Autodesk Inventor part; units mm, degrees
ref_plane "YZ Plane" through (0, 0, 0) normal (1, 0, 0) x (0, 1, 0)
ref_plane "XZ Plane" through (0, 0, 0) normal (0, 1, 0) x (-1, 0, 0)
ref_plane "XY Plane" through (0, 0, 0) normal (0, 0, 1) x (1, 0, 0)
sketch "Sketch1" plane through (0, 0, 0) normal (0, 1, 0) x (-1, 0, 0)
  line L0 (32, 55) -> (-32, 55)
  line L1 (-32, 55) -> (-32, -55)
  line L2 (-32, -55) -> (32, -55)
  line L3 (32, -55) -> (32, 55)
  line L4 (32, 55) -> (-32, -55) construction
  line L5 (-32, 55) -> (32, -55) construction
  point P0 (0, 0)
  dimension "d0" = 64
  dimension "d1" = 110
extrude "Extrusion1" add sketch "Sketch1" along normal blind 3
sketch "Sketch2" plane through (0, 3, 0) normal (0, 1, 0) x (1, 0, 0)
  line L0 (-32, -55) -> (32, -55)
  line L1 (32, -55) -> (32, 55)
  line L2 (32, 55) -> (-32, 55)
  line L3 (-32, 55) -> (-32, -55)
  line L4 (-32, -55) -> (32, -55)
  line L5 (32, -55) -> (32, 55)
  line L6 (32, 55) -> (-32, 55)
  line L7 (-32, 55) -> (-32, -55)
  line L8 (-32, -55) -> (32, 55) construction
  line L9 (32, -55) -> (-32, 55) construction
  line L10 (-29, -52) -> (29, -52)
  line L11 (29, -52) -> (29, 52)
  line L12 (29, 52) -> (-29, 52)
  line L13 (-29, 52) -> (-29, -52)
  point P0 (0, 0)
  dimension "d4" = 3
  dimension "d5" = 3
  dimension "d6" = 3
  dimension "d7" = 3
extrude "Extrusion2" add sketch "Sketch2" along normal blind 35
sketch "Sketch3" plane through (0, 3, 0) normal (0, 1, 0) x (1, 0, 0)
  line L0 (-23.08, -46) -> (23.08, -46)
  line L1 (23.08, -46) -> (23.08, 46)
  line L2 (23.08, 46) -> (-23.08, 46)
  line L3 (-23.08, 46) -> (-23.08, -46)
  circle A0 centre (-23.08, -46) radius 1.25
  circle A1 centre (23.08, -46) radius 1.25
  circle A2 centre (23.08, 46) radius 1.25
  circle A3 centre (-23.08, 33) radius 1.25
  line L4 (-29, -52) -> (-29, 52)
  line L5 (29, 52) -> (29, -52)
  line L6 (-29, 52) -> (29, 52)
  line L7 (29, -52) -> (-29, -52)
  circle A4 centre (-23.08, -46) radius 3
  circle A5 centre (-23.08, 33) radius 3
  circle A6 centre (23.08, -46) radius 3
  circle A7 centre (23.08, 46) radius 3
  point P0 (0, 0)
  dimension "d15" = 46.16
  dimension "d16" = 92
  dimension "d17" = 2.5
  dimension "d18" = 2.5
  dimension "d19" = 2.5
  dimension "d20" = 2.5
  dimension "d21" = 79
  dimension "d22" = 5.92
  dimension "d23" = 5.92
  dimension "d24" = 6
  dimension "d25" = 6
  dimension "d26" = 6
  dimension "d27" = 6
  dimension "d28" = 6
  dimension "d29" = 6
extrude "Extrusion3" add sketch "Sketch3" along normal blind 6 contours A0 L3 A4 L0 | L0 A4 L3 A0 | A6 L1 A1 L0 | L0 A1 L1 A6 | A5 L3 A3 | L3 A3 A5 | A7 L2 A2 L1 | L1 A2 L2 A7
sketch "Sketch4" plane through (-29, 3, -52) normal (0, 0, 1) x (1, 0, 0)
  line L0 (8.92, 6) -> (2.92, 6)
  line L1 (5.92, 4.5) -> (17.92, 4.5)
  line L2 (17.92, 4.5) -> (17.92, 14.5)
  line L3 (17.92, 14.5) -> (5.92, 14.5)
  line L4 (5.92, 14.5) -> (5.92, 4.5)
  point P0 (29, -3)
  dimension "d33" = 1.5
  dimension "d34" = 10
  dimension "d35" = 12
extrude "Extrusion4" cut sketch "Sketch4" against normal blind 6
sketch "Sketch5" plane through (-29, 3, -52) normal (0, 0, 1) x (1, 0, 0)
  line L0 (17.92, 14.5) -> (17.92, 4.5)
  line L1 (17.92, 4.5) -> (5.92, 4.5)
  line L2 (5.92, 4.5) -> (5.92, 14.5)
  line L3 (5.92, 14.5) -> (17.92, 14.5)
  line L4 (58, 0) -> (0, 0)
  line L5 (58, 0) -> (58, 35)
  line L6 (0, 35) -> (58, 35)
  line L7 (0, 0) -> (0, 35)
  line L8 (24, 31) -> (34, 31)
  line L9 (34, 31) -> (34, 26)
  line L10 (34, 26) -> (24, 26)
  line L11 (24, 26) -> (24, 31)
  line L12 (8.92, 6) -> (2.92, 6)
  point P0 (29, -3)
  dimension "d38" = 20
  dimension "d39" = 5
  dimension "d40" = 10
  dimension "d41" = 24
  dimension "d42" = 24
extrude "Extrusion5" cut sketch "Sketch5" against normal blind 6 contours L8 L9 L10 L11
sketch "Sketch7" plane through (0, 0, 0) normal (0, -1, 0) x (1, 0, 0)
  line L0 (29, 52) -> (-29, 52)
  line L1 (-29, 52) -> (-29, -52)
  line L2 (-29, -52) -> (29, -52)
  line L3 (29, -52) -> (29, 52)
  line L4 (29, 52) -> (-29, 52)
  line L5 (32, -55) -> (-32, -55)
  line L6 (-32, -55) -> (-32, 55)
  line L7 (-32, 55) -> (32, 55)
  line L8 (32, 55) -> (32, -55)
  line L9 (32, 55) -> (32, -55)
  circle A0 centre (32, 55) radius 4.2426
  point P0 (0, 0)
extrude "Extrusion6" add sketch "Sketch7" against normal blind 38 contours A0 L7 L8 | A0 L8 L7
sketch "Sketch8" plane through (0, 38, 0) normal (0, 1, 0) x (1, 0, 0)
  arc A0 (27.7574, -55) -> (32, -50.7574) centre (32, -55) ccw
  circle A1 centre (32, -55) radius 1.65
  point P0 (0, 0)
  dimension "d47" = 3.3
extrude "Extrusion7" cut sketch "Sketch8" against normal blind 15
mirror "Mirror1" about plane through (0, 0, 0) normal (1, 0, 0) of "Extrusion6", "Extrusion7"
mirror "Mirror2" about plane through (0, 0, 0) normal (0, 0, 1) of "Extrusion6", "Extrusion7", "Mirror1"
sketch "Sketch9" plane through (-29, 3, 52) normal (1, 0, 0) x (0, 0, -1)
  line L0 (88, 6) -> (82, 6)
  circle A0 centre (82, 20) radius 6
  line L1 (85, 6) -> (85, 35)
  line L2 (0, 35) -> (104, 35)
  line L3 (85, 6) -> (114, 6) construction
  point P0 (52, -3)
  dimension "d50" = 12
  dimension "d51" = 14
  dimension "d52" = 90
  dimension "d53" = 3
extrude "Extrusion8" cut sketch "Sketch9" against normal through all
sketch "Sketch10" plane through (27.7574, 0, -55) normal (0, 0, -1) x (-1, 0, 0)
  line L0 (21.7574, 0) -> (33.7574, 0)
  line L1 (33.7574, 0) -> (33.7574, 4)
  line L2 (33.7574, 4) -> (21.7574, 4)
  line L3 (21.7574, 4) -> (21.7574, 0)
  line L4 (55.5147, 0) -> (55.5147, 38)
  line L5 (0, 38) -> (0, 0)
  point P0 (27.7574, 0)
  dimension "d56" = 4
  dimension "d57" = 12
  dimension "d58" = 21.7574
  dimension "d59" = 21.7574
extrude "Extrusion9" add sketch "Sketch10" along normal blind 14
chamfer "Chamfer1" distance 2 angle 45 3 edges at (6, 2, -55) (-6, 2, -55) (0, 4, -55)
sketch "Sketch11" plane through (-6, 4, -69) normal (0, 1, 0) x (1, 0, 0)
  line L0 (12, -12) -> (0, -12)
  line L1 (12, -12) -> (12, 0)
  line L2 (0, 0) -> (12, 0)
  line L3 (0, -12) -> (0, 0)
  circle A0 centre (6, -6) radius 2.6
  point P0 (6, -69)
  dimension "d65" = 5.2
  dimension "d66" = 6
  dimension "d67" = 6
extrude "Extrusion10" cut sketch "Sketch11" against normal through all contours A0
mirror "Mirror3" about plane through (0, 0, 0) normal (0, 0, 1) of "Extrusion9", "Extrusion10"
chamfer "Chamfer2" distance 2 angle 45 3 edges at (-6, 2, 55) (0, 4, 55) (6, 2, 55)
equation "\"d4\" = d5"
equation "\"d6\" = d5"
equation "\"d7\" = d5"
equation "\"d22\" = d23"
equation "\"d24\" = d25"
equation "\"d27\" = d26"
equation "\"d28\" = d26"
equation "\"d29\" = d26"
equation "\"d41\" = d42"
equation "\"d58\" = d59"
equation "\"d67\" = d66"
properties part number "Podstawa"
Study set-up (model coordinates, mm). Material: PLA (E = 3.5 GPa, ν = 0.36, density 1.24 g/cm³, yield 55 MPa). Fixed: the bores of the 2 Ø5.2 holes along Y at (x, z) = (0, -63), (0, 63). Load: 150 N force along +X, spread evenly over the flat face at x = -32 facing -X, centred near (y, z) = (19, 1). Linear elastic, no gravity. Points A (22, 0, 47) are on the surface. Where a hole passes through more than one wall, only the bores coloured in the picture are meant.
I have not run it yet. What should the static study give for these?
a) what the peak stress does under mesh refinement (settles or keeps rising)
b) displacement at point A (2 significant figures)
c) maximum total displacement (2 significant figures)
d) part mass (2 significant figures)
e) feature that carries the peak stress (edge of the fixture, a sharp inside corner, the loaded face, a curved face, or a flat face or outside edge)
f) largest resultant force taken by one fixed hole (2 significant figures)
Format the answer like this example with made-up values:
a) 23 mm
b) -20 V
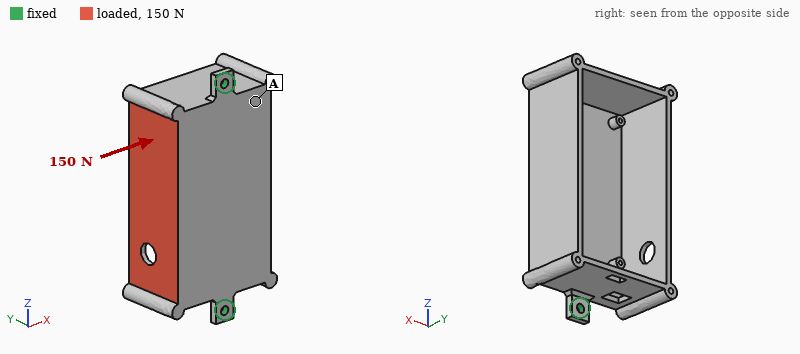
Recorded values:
a) keeps rising
b) 0.48 mm
c) 1.9 mm
d) 79 g
e) edge of the fixture
f) 77 N
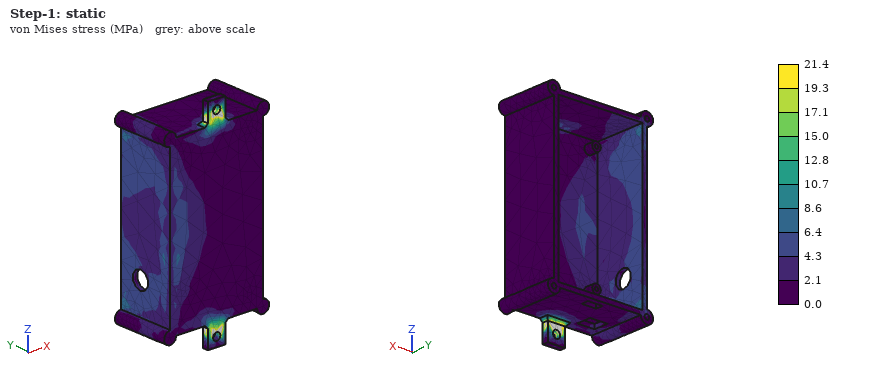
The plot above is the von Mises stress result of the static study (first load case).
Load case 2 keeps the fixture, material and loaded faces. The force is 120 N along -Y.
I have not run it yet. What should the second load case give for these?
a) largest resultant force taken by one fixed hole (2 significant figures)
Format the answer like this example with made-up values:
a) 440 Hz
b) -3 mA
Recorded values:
a) 61 N
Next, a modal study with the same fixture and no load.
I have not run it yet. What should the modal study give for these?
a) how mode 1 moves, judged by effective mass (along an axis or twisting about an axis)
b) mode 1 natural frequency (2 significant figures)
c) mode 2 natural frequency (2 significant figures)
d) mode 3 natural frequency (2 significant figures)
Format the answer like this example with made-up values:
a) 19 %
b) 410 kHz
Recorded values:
a) along X
b) 200 Hz
c) 370 Hz
d) 670 Hz
